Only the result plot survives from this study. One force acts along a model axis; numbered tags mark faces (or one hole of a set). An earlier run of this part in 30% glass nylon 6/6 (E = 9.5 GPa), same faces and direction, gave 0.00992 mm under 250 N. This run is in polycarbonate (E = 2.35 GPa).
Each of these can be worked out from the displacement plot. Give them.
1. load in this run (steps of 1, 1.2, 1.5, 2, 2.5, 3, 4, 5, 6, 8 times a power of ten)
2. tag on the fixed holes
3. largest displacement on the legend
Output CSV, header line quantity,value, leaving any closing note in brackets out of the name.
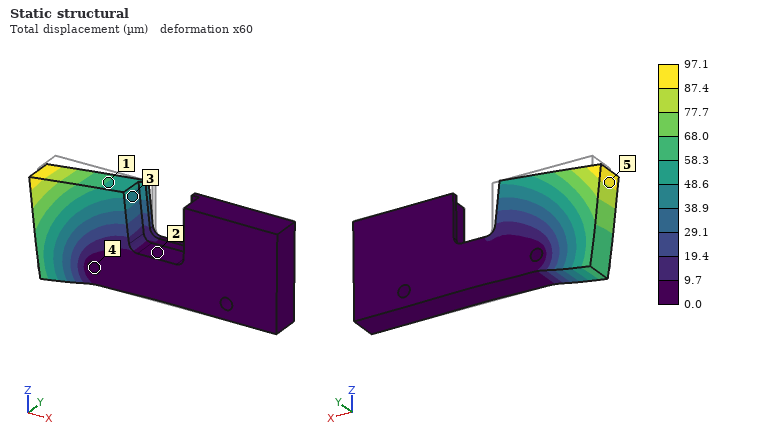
quantity,value
load in this run,600 N
tag on the fixed holes,4
largest displacement on the legend,97.1 µm
